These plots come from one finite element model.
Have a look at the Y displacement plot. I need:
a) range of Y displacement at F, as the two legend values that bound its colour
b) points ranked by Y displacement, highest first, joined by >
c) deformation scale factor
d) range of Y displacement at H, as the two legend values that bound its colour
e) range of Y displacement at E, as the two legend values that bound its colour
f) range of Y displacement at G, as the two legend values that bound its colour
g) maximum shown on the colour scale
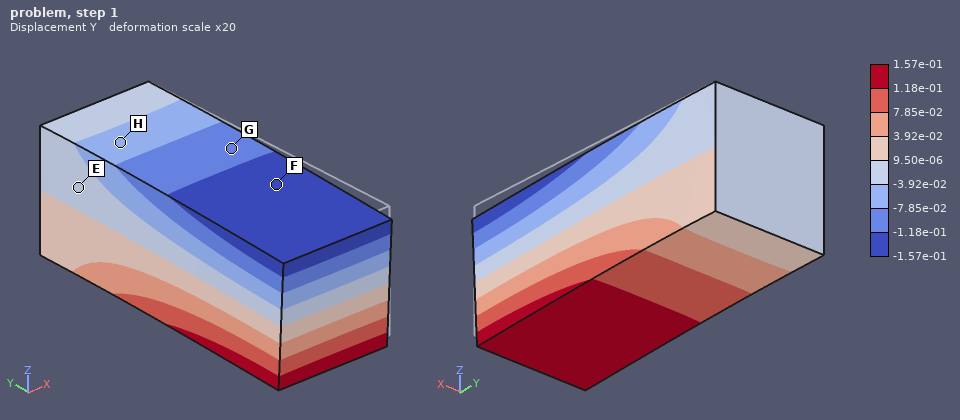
-1.57e-01 to -1.18e-01
E > H > G > F
20
-7.85e-02 to -3.92e-02
-3.92e-02 to 9.50e-06
-1.18e-01 to -7.85e-02
1.57e-01
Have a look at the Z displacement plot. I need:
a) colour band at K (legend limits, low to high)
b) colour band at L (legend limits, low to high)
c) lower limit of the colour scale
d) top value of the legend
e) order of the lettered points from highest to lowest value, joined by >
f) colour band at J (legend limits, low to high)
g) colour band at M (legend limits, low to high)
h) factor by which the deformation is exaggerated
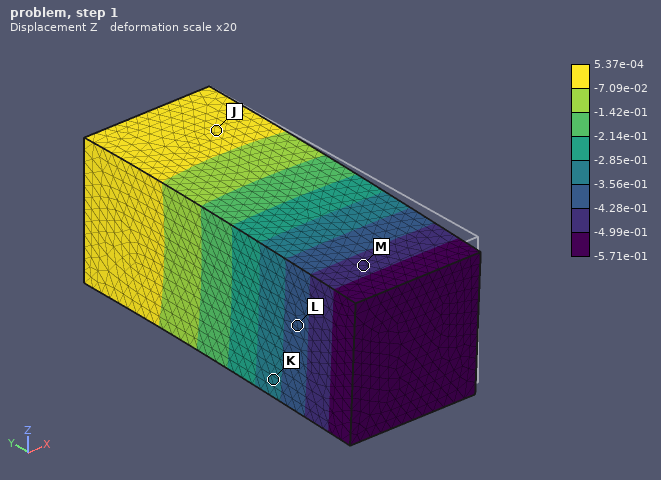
-3.56e-01 to -2.85e-01
-4.28e-01 to -3.56e-01
-5.71e-01
5.37e-04
J > K > L > M
-7.09e-02 to 5.37e-04
-4.99e-01 to -4.28e-01
20
